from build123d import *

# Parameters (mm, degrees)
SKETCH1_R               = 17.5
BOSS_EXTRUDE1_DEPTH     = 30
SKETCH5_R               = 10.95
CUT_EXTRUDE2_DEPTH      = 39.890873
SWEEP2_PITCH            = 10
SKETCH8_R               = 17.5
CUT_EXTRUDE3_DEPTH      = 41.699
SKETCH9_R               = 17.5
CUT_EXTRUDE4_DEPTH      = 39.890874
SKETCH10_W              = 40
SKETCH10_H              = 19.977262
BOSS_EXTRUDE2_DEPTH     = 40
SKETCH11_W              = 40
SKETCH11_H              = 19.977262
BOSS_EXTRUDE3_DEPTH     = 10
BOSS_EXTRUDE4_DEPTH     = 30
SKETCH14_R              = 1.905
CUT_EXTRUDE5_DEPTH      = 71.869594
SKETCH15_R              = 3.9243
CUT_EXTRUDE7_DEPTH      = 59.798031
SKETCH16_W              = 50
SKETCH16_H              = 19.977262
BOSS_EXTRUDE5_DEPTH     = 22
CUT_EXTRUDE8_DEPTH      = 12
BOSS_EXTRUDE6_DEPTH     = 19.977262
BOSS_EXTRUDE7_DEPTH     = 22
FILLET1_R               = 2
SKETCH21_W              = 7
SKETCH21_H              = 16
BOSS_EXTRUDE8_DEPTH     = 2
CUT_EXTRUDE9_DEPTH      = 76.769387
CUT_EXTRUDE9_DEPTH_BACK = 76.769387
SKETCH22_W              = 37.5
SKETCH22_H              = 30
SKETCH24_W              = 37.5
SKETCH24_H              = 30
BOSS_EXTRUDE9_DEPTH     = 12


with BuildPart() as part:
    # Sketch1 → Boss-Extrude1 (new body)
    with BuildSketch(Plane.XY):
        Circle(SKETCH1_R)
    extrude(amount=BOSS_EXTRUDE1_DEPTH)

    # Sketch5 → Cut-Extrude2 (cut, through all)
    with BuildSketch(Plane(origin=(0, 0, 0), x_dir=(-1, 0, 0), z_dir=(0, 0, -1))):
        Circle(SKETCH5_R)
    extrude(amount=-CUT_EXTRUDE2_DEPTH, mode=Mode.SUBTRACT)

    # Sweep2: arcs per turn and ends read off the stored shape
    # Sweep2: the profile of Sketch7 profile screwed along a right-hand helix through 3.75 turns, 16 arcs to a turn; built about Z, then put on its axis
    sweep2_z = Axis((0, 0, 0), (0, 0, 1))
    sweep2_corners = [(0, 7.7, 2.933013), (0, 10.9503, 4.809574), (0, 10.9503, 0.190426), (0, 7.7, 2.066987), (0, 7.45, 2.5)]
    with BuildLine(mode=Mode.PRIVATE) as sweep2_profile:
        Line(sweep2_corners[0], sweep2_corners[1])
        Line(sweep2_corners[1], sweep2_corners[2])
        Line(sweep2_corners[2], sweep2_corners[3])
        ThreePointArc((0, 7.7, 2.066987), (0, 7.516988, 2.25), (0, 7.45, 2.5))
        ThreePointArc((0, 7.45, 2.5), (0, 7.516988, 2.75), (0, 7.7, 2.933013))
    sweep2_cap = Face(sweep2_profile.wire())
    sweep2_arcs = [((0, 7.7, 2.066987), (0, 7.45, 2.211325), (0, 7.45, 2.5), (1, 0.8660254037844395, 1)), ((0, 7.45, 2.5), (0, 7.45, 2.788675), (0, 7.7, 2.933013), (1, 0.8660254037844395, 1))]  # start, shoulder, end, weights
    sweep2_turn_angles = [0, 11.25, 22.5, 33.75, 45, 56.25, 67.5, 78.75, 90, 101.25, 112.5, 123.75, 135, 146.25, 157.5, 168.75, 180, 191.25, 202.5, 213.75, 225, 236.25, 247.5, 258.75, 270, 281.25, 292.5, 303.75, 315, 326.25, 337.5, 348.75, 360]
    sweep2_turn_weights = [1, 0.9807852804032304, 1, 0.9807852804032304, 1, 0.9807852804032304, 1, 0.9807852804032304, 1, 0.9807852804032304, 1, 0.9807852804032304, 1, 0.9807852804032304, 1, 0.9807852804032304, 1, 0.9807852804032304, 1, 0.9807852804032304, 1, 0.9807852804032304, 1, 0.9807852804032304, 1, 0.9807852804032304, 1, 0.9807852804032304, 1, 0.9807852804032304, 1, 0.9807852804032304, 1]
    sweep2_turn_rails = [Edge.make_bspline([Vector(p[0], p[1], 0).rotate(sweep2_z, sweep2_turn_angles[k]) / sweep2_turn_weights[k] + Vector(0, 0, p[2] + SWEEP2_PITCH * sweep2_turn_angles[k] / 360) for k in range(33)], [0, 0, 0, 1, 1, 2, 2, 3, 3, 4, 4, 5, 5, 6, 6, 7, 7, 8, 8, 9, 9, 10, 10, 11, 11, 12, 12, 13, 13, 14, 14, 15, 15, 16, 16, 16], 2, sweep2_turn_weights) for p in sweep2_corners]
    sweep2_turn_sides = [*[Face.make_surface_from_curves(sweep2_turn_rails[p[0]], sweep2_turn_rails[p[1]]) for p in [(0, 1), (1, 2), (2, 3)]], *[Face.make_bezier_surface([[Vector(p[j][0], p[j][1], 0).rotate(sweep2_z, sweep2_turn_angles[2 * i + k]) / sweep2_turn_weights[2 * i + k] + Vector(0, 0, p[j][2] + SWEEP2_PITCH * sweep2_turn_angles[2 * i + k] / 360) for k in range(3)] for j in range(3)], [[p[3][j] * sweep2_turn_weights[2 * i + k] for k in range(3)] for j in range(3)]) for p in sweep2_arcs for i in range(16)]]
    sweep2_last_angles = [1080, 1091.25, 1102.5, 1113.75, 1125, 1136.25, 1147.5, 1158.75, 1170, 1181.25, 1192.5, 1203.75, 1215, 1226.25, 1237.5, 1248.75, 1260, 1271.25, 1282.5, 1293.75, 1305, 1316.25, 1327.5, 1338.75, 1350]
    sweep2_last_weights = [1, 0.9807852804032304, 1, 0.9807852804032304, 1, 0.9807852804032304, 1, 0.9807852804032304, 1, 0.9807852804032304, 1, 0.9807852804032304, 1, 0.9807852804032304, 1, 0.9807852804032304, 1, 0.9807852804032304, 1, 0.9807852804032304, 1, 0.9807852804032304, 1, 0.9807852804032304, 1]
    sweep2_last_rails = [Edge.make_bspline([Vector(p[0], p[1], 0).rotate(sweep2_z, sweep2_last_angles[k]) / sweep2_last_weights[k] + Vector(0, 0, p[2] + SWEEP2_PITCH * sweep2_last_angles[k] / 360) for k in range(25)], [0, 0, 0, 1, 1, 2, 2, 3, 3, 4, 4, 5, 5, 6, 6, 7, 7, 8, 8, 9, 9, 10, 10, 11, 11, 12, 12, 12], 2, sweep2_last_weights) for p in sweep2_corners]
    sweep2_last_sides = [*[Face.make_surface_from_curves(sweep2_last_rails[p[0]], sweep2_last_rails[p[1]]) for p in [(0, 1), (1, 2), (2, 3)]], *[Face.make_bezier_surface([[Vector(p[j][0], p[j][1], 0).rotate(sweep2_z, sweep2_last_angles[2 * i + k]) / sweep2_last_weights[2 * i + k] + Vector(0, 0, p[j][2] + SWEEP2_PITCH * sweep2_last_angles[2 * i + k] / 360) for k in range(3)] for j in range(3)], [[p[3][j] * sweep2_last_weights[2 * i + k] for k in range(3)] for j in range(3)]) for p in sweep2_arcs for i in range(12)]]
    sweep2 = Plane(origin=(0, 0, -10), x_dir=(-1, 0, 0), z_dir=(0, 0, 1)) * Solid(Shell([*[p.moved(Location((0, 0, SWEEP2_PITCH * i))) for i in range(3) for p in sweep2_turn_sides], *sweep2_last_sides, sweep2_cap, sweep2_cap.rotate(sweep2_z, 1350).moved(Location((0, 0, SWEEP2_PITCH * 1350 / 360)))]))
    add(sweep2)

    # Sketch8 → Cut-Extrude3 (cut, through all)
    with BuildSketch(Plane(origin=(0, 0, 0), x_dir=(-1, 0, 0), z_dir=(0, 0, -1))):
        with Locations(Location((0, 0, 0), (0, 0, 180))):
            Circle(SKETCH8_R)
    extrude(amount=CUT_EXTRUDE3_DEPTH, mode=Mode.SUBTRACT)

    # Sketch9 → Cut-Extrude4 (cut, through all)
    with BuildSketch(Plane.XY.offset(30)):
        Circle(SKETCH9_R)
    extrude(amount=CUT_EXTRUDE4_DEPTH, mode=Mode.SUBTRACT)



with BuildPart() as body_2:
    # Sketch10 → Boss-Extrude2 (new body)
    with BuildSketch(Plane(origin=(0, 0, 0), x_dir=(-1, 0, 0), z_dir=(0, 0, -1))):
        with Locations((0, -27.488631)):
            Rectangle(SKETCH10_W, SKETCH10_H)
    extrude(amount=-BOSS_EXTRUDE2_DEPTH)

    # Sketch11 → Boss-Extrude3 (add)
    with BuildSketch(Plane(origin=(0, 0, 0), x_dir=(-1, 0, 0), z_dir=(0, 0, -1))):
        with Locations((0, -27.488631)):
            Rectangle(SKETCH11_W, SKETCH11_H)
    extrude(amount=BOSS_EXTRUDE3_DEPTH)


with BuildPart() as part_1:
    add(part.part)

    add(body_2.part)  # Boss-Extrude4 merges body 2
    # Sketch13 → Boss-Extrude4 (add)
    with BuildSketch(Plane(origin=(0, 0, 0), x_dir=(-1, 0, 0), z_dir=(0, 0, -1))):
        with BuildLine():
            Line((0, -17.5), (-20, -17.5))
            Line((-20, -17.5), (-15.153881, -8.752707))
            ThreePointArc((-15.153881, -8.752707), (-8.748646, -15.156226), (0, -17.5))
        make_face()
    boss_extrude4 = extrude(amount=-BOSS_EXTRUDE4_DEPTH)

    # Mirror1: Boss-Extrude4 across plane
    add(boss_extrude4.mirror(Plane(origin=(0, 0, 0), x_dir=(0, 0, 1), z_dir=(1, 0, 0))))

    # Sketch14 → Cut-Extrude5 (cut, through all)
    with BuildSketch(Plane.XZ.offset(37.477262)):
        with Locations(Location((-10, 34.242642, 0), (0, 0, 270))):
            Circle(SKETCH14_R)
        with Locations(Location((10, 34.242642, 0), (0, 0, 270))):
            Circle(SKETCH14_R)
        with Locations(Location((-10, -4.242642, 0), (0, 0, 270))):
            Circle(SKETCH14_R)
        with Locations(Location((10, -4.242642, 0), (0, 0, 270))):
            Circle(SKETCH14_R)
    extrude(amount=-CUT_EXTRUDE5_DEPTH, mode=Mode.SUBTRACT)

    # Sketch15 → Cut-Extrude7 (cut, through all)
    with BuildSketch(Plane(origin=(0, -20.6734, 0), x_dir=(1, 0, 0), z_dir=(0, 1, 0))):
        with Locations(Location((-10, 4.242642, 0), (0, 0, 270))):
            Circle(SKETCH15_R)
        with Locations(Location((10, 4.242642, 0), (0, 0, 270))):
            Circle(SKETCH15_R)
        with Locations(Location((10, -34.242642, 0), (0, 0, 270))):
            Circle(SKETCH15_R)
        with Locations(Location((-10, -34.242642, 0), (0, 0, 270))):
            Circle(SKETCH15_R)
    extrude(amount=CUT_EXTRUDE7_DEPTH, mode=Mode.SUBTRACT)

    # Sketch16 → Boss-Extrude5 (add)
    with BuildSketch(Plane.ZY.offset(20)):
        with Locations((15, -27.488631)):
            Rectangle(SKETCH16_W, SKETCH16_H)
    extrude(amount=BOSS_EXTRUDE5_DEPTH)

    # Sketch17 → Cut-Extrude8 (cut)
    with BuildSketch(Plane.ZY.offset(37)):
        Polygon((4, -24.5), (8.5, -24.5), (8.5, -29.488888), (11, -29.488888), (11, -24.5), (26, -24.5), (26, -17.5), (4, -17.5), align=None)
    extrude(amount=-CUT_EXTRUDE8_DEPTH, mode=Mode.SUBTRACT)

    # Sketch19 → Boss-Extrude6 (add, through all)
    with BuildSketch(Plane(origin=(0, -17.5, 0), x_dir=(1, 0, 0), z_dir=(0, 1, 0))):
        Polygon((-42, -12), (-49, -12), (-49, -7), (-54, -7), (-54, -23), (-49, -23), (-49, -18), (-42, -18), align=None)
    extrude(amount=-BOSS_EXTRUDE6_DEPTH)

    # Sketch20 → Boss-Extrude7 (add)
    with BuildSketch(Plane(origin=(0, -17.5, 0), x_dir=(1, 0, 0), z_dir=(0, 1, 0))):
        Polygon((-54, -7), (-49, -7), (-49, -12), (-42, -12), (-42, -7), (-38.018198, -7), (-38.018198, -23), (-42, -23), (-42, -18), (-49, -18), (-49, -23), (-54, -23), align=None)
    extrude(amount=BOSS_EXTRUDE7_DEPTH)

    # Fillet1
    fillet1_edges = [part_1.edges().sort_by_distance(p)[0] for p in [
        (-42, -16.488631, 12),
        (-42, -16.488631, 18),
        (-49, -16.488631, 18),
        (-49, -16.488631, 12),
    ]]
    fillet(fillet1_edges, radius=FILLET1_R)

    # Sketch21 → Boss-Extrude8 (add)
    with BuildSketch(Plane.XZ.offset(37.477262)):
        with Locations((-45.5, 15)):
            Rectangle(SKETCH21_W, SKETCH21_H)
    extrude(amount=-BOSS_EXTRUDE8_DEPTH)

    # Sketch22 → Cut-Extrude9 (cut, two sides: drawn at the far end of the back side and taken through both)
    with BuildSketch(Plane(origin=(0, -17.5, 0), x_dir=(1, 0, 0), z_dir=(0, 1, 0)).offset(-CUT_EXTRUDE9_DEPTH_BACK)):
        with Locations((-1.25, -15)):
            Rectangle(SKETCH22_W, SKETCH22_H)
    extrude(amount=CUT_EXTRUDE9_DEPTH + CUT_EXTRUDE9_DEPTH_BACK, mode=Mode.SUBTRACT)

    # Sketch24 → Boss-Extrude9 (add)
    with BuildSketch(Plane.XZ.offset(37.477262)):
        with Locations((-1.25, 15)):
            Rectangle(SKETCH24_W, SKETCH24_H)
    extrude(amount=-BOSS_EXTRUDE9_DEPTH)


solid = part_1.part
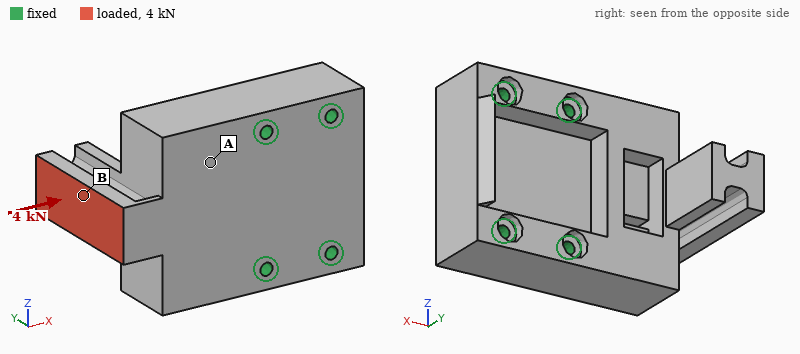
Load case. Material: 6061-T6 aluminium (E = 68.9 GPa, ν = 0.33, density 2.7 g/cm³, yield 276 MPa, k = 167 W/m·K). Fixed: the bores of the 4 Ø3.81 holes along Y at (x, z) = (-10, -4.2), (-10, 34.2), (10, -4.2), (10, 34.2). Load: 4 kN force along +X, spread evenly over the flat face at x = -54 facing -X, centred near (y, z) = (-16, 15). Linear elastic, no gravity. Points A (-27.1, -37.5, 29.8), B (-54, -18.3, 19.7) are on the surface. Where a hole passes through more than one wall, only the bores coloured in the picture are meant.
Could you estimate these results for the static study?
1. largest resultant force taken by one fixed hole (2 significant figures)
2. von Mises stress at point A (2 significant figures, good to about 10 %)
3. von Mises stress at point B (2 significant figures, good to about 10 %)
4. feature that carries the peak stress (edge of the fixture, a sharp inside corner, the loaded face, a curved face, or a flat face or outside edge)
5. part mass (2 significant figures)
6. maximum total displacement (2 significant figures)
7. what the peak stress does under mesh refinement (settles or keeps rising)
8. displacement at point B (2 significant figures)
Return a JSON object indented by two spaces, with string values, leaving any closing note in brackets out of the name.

{
  "largest resultant force taken by one fixed hole": "1.8 kN",
  "von Mises stress at point A": "16 MPa",
  "von Mises stress at point B": "44 MPa",
  "feature that carries the peak stress": "a sharp inside corner",
  "part mass": "150 g",
  "maximum total displacement": "0.20 mm",
  "what the peak stress does under mesh refinement": "keeps rising",
  "displacement at point B": "0.11 mm"
}
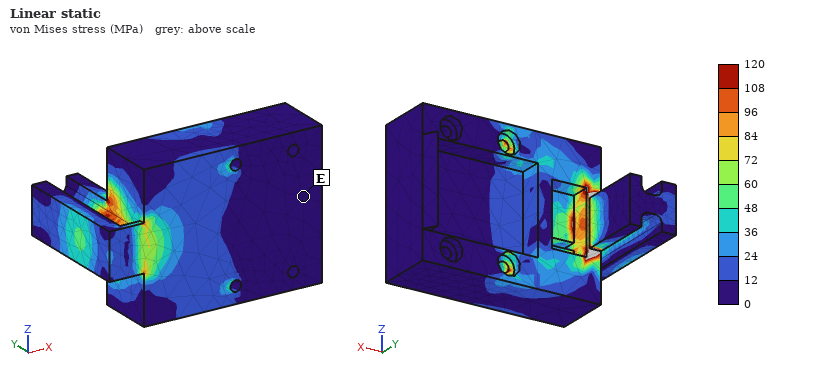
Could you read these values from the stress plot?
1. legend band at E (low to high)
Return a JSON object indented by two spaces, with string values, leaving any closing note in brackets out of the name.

{
  "legend band at E": "0 to 12 MPa"
}
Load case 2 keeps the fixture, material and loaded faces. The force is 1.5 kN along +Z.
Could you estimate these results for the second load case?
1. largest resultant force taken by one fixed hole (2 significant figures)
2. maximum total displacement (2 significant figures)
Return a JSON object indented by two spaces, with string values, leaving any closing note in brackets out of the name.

{
  "largest resultant force taken by one fixed hole": "1.7 kN",
  "maximum total displacement": "0.10 mm"
}
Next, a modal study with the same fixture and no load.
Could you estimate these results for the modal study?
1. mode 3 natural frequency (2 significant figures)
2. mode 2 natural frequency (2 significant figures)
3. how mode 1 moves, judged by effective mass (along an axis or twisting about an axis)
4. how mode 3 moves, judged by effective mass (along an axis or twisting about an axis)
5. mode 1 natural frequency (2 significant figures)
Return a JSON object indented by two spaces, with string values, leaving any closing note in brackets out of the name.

{
  "mode 3 natural frequency": "9200 Hz",
  "mode 2 natural frequency": "7000 Hz",
  "how mode 1 moves, judged by effective mass": "along Y",
  "how mode 3 moves, judged by effective mass": "along Y",
  "mode 1 natural frequency": "4700 Hz"
}
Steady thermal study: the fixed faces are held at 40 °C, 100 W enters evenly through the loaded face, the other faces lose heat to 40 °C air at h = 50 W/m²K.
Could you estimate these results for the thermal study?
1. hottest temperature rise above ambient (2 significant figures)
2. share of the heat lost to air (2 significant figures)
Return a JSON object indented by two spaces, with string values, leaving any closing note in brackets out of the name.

{
  "hottest temperature rise above ambient": "81 K",
  "share of the heat lost to air": "12 %"
}
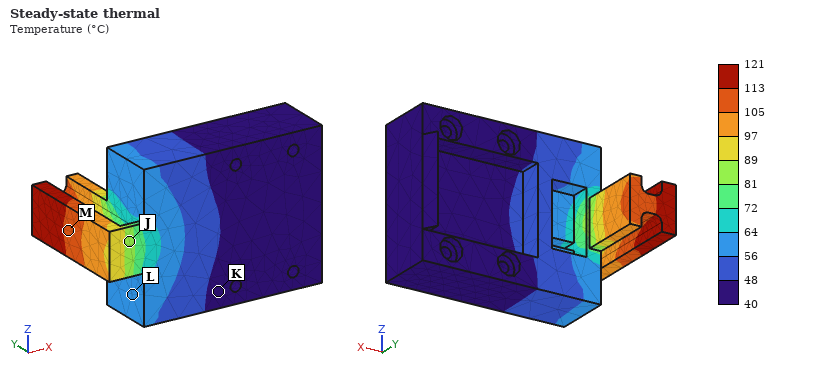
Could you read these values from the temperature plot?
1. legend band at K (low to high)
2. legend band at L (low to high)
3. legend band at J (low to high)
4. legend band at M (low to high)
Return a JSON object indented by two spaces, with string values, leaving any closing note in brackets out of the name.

{
  "legend band at K": "40 to 48 °C",
  "legend band at L": "56 to 64 °C",
  "legend band at J": "81 to 89 °C",
  "legend band at M": "105 to 113 °C"
}
